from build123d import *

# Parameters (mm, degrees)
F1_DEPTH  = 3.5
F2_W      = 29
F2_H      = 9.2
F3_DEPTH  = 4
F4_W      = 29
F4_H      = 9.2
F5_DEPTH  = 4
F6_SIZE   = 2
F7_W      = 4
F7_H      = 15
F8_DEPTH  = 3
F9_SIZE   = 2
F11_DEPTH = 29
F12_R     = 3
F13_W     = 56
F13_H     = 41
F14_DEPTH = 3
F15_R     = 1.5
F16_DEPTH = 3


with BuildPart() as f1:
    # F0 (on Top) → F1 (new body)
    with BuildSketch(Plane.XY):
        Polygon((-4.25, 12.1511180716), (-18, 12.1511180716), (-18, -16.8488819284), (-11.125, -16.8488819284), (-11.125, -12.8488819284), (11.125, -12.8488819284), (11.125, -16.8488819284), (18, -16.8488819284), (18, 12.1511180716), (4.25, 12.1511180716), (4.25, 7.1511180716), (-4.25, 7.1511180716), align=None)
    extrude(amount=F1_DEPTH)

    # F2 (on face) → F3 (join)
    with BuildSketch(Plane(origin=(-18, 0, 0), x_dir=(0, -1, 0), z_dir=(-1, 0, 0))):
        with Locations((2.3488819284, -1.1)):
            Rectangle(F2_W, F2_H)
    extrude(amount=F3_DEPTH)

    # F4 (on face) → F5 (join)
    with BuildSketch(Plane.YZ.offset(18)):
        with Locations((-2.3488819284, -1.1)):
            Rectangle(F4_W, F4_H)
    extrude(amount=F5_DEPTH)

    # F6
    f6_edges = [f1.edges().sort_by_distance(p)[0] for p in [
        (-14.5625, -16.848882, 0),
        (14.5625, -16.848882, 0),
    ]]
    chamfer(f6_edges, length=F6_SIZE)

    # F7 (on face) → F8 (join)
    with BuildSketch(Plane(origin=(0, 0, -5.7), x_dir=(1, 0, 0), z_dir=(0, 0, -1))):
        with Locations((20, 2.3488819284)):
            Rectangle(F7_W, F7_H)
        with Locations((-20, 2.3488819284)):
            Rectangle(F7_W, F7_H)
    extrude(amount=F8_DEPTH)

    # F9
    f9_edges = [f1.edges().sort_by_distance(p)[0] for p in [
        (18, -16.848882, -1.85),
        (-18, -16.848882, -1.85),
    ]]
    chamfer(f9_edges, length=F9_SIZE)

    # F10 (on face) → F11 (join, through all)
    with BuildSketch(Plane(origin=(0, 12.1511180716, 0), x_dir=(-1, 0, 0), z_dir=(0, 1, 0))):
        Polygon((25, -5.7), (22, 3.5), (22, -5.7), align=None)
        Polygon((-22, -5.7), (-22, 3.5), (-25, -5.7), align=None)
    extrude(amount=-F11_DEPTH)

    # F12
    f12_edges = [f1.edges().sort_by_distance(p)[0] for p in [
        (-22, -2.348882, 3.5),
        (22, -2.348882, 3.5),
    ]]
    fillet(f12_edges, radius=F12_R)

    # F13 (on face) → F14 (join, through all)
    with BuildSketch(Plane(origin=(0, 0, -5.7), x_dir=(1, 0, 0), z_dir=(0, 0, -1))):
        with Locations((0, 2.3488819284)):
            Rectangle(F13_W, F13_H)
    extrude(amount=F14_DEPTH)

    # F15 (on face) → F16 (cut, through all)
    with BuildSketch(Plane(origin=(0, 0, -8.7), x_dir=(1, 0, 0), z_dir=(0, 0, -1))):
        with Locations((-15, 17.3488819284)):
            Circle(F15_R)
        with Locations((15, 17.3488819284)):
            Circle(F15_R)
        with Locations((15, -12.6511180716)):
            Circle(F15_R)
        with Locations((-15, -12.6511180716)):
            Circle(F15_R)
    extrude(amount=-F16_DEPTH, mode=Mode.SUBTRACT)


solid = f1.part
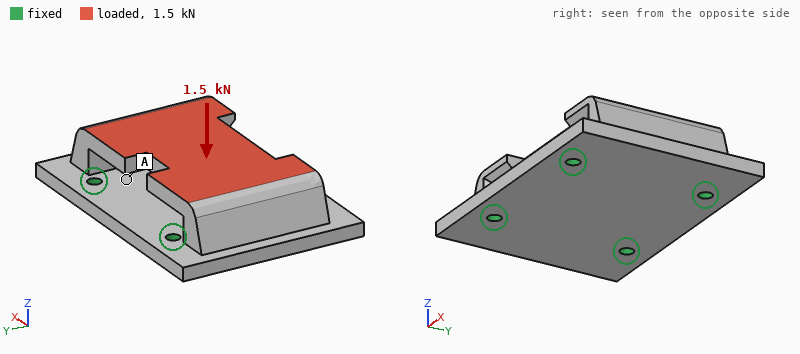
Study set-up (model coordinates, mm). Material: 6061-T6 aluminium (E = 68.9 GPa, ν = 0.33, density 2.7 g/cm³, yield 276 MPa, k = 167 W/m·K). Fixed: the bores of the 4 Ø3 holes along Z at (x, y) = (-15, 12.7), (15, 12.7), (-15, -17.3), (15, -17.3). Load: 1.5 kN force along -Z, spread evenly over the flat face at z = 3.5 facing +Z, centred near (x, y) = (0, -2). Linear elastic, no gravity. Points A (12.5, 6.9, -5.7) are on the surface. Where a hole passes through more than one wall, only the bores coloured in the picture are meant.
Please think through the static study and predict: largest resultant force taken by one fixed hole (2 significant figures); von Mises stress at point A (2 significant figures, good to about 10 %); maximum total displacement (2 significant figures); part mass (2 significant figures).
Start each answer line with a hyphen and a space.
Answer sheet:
- 400 N
- 12 MPa
- 53 µm
- 35 g
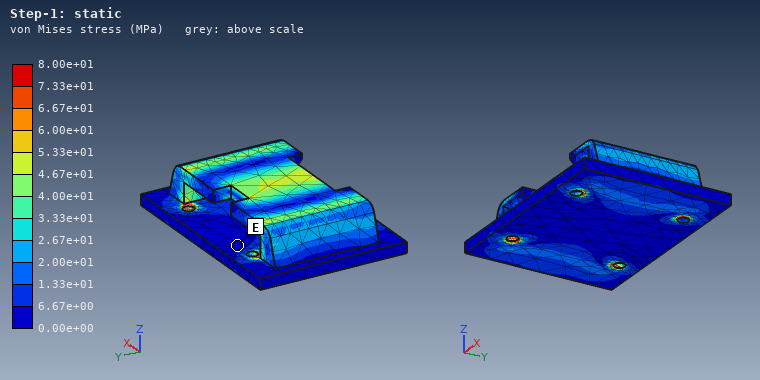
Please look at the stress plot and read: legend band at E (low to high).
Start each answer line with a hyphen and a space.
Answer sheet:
- 0.00e+00 to 6.67e+00 MPa
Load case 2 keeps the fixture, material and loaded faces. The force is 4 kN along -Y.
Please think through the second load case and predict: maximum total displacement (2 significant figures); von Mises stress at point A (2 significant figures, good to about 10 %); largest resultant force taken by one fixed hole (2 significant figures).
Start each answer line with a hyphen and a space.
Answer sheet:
- 56 µm
- 26 MPa
- 1.3 kN
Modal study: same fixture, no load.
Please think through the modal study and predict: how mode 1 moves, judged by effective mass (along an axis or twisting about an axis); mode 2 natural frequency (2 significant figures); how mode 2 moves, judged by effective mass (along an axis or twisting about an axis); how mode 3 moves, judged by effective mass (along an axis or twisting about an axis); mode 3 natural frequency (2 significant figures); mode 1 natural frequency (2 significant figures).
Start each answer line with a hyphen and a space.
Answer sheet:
- along X
- 9900 Hz
- along Z
- along Z
- 14 kHz
- 7900 Hz
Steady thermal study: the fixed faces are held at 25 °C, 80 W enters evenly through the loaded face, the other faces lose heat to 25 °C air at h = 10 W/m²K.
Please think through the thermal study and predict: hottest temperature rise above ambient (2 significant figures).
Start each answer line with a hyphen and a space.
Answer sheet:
- 53 K
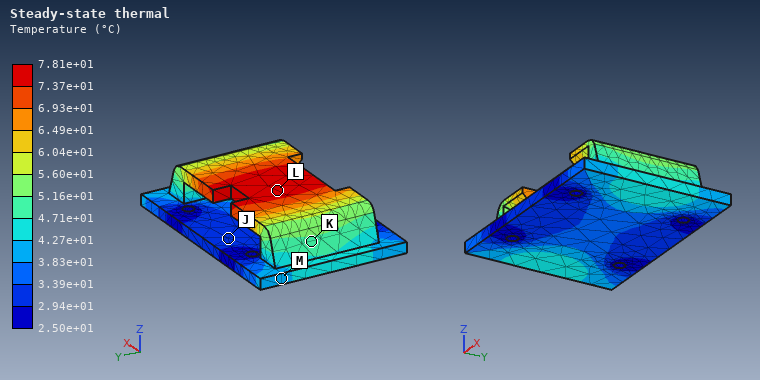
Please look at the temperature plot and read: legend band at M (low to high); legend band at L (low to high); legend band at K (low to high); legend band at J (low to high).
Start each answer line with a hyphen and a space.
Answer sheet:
- 3.83e+01 to 4.27e+01 °C
- 7.37e+01 to 7.81e+01 °C
- 4.71e+01 to 5.16e+01 °C
- 2.94e+01 to 3.39e+01 °C
